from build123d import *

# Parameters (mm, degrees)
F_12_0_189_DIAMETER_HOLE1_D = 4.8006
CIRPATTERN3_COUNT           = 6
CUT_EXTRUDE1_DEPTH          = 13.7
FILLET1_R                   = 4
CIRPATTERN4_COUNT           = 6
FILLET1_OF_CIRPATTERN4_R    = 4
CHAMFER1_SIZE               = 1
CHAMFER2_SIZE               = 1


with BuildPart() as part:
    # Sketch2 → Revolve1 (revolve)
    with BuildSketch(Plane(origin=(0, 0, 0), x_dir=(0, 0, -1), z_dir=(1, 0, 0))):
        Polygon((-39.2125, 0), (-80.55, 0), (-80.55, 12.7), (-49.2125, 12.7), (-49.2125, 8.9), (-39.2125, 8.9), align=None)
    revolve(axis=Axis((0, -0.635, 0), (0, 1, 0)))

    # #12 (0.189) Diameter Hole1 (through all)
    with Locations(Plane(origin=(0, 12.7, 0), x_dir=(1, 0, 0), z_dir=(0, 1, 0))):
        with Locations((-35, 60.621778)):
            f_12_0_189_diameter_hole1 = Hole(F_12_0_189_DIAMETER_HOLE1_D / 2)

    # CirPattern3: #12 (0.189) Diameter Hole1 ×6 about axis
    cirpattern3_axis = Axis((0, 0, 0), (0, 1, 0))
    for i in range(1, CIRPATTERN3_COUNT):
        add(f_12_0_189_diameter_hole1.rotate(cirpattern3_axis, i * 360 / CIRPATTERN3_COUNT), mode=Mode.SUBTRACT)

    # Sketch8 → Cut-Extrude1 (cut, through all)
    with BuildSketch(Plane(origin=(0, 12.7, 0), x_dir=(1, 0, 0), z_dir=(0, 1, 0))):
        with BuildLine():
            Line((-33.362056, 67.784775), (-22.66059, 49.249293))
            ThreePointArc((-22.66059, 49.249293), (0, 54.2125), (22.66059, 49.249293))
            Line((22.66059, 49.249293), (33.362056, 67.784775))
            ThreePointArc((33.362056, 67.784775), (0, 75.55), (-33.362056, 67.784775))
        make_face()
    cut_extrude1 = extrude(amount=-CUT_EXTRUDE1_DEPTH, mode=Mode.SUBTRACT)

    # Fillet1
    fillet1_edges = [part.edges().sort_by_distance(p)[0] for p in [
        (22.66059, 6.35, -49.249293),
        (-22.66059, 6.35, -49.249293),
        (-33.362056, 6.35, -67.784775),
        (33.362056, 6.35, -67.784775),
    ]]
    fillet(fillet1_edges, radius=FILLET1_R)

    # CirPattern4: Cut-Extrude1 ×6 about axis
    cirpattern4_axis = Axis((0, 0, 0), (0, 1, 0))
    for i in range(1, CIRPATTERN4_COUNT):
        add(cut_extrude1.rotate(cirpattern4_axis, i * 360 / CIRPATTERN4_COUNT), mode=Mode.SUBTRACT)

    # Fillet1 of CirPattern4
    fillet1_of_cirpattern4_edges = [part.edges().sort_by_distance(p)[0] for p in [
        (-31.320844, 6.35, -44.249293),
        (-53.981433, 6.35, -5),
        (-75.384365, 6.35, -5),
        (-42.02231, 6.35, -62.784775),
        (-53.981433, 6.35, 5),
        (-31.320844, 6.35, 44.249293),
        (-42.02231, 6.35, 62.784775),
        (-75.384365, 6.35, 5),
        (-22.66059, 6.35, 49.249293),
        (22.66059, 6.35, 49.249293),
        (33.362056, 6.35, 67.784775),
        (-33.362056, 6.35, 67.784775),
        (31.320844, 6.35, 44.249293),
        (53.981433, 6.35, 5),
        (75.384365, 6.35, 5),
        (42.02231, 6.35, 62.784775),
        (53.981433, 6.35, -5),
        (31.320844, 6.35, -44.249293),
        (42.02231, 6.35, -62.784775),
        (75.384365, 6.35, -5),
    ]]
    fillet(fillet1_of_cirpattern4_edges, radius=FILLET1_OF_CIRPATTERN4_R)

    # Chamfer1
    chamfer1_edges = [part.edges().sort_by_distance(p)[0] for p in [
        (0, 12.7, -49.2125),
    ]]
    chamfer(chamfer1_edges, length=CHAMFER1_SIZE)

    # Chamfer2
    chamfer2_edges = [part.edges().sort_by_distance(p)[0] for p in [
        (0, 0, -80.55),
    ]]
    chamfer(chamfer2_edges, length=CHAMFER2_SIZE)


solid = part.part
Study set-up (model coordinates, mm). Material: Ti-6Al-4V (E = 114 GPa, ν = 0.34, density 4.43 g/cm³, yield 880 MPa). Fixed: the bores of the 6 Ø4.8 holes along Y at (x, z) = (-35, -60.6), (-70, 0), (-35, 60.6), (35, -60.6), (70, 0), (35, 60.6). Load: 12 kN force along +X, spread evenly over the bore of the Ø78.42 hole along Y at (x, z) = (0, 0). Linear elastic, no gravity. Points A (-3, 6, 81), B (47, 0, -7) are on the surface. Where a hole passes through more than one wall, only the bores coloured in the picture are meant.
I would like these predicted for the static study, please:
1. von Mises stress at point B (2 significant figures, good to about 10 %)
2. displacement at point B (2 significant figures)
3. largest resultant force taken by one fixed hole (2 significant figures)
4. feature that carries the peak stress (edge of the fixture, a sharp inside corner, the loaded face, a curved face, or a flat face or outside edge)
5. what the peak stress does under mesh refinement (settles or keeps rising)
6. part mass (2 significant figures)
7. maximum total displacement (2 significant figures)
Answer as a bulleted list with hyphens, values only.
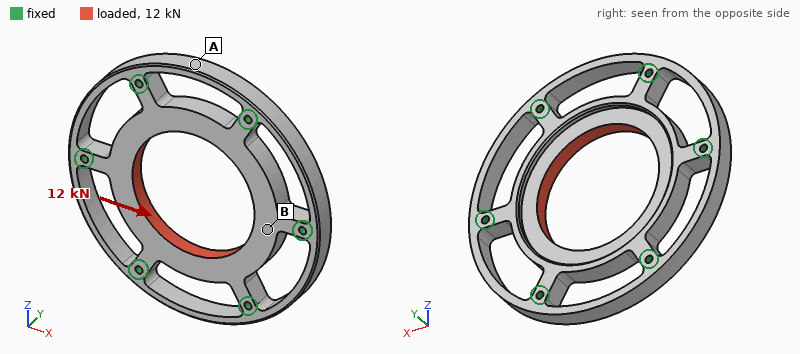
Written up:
- 19 MPa
- 6.8 µm
- 3.2 kN
- edge of the fixture
- keeps rising
- 410 g
- 12 µm
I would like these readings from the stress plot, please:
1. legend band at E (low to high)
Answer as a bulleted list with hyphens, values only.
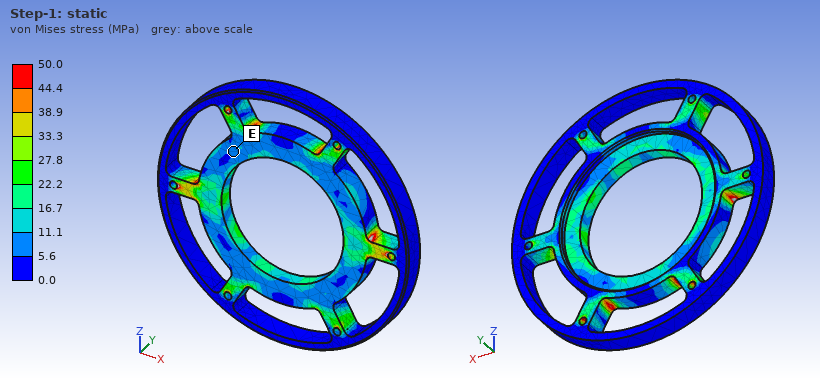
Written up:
- 5.6 to 11.1 MPa
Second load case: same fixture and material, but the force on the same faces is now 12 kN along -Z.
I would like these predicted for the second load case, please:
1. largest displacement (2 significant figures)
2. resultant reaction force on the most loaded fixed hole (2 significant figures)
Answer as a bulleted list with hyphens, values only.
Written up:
- 13 µm
- 2.8 kN
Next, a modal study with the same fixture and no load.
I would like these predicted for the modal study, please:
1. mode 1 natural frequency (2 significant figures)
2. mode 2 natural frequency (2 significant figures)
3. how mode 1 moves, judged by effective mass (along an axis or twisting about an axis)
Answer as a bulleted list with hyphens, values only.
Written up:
- 6300 Hz
- 7100 Hz
- along Y
